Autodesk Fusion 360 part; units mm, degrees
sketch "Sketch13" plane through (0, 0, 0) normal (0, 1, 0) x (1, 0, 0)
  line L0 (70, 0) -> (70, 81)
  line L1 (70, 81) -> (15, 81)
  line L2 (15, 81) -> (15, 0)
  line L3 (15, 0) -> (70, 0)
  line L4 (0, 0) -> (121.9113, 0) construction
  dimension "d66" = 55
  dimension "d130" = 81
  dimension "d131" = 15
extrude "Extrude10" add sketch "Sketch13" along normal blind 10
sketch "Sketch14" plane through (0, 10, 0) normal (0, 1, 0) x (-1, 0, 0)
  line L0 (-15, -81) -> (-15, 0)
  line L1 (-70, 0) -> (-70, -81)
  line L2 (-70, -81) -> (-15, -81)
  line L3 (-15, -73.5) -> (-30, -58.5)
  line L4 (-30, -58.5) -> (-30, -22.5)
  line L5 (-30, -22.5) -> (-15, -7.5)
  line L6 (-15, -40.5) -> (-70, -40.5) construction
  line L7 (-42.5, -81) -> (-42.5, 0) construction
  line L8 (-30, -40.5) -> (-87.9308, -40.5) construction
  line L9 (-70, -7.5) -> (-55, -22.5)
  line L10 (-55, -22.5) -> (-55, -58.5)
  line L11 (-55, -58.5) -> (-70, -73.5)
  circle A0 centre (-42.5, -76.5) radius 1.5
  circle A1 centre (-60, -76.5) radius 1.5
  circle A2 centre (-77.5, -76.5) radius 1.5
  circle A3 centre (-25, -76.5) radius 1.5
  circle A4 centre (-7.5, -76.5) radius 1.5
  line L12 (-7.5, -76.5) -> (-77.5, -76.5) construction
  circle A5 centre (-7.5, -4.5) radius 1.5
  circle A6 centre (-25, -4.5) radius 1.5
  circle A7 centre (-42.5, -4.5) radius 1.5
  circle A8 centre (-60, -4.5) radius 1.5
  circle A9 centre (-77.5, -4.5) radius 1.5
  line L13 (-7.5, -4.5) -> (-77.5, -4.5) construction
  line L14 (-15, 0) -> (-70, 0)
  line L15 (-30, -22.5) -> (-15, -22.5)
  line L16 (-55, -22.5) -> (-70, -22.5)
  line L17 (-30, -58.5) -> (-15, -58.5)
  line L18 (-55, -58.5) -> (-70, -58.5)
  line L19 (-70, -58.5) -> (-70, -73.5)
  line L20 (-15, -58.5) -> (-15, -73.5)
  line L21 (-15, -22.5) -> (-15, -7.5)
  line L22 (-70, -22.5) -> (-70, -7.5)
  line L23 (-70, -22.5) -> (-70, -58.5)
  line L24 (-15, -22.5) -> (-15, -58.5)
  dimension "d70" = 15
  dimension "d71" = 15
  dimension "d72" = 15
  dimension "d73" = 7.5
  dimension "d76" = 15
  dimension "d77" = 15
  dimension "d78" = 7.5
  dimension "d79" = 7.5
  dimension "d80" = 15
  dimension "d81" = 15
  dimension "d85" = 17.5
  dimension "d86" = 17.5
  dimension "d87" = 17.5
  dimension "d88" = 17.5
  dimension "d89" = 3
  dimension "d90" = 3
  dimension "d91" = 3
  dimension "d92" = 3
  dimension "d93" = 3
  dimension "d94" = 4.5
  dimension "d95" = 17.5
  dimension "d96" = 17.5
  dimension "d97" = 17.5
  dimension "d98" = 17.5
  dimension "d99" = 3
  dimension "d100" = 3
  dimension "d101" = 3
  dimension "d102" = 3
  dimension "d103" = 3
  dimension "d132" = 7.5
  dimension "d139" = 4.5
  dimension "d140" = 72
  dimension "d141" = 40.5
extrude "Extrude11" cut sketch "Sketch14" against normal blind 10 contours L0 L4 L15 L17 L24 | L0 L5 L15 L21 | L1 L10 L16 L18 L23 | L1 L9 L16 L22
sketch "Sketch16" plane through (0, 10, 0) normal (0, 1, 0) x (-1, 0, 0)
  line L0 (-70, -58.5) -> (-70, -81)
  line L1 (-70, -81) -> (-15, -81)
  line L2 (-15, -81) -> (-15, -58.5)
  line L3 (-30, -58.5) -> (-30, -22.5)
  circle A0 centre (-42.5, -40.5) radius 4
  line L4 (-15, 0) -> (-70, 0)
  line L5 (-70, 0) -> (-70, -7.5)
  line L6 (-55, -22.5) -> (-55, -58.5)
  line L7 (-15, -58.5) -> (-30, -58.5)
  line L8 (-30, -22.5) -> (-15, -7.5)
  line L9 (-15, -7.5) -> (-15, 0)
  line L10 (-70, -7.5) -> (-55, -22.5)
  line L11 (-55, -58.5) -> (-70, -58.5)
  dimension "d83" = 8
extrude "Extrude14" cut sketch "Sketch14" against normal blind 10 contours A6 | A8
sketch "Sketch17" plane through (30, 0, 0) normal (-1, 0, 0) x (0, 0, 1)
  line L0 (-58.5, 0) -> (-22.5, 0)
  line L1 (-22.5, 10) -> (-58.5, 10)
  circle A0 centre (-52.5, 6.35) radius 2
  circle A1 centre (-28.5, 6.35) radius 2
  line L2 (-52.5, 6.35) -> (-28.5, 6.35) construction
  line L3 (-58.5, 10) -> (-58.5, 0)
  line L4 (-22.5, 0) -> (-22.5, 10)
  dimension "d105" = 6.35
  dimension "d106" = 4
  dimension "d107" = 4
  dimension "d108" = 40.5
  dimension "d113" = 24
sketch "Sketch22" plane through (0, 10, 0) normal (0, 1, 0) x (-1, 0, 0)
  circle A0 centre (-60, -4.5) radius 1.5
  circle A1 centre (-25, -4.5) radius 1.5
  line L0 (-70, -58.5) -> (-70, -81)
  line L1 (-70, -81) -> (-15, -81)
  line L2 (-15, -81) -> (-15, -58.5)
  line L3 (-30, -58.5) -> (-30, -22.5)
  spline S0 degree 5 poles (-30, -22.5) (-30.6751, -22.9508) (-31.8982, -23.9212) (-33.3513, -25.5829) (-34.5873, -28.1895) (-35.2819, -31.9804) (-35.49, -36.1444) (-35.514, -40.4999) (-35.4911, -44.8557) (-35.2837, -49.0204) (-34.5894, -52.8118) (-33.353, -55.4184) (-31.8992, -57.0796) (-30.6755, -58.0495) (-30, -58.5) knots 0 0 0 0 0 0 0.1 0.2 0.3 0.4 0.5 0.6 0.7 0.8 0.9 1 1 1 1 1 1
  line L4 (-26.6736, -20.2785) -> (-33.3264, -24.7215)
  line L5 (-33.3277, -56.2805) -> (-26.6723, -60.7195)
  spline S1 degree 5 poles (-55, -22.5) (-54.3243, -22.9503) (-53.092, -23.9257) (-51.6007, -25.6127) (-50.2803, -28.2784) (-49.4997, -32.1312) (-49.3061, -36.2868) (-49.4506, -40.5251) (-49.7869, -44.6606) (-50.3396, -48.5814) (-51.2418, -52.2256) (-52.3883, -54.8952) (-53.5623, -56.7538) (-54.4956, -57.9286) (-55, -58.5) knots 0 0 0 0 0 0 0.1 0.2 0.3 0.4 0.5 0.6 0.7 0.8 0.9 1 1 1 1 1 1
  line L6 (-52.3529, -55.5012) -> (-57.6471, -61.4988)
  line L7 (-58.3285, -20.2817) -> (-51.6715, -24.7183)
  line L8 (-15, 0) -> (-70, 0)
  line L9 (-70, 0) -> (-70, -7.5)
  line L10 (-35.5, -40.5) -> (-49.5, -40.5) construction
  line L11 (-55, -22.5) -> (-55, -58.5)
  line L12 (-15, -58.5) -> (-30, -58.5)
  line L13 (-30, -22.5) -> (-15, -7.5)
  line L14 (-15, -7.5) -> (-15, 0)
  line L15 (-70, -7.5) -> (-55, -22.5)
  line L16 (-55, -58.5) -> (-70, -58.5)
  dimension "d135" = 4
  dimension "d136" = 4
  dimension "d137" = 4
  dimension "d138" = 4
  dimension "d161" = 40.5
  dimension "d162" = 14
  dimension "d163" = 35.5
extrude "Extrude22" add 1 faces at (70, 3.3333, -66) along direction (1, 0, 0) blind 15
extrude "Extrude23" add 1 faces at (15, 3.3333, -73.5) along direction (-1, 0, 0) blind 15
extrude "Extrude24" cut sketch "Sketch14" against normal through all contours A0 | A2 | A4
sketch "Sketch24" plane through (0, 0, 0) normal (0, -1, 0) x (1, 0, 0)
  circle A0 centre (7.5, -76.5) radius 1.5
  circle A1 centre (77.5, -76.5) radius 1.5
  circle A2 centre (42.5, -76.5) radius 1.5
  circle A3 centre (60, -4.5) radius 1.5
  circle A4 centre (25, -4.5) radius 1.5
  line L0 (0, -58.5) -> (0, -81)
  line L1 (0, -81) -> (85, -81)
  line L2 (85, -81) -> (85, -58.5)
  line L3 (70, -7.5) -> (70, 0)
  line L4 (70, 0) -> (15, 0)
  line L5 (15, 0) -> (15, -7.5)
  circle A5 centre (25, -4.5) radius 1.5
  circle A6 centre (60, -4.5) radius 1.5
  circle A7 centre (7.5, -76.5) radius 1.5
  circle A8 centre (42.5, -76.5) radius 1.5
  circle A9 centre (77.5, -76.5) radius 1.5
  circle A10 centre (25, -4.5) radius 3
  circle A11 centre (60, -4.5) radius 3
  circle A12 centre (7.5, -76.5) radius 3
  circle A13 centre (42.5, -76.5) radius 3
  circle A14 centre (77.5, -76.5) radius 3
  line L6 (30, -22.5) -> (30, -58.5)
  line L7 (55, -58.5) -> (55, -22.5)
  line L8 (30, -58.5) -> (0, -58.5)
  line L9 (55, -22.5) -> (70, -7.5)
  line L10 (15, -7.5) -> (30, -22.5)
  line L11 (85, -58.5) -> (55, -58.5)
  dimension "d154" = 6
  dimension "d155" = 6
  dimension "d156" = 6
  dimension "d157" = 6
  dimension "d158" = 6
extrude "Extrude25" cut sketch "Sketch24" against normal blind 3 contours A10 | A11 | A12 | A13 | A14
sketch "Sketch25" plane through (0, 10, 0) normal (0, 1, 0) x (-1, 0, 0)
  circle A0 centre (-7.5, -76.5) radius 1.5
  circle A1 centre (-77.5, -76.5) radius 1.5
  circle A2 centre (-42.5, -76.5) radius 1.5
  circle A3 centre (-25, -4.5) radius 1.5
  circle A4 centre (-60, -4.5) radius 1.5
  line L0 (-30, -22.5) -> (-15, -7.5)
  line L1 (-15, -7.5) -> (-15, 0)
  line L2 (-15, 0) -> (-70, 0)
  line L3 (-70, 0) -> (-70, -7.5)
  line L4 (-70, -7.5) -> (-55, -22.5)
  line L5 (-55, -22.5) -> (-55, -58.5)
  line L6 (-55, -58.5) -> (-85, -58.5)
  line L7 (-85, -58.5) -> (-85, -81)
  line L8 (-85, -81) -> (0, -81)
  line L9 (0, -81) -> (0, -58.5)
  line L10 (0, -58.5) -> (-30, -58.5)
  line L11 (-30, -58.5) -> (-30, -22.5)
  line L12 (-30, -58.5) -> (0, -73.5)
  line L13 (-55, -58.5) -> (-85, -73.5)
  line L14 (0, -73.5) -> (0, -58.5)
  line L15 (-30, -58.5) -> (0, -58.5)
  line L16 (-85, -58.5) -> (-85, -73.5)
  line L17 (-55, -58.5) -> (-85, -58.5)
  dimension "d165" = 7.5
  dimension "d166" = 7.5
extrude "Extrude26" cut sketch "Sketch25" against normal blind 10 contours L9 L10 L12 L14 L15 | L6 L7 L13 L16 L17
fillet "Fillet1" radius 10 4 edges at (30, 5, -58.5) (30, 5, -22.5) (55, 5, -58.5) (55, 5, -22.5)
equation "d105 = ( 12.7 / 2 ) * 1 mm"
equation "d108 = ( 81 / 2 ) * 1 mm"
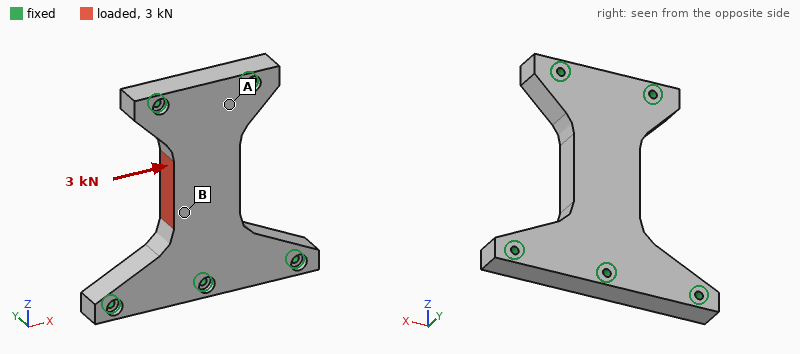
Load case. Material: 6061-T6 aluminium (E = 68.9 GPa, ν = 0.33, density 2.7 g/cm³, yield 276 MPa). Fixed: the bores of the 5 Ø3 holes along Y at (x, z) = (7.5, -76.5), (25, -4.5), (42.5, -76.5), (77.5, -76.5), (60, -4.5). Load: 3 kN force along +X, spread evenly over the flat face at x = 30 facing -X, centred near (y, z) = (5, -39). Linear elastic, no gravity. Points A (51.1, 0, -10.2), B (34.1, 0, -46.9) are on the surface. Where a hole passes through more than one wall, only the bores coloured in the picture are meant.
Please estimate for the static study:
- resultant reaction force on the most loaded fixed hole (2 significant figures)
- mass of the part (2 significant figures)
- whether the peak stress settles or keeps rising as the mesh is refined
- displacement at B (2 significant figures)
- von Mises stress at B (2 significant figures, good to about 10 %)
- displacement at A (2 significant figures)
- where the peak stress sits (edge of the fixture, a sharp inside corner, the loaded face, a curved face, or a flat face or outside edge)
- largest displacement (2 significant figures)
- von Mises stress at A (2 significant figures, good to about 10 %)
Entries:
1.2 kN
90 g
keeps rising
8.6 µm
11 MPa
1.8 µm
edge of the fixture
10 µm
5.3 MPa
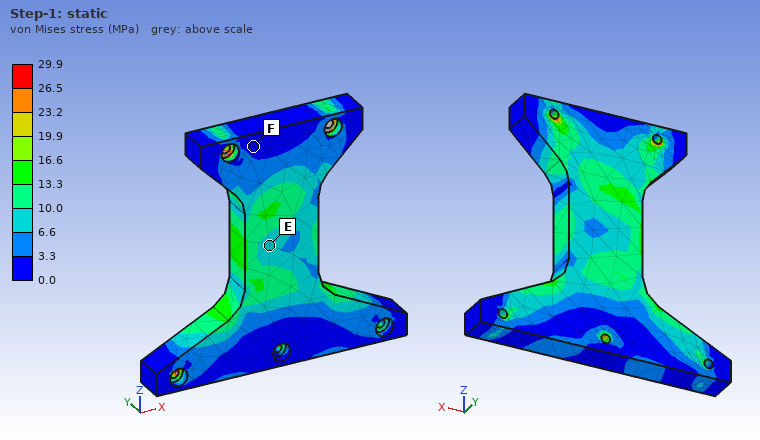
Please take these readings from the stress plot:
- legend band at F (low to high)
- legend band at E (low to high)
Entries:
0.0 to 3.3 MPa
6.6 to 10.0 MPa
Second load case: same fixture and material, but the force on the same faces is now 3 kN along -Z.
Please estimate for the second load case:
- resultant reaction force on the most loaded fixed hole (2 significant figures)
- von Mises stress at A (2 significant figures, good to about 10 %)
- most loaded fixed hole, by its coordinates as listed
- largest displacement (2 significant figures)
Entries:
1.2 kN
5.9 MPa
(42.5, -76.5)
7.2 µm
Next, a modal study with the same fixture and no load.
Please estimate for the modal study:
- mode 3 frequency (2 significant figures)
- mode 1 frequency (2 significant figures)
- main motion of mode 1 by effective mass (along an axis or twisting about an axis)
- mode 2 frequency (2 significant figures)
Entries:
16 kHz
7000 Hz
along Y
16 kHz
